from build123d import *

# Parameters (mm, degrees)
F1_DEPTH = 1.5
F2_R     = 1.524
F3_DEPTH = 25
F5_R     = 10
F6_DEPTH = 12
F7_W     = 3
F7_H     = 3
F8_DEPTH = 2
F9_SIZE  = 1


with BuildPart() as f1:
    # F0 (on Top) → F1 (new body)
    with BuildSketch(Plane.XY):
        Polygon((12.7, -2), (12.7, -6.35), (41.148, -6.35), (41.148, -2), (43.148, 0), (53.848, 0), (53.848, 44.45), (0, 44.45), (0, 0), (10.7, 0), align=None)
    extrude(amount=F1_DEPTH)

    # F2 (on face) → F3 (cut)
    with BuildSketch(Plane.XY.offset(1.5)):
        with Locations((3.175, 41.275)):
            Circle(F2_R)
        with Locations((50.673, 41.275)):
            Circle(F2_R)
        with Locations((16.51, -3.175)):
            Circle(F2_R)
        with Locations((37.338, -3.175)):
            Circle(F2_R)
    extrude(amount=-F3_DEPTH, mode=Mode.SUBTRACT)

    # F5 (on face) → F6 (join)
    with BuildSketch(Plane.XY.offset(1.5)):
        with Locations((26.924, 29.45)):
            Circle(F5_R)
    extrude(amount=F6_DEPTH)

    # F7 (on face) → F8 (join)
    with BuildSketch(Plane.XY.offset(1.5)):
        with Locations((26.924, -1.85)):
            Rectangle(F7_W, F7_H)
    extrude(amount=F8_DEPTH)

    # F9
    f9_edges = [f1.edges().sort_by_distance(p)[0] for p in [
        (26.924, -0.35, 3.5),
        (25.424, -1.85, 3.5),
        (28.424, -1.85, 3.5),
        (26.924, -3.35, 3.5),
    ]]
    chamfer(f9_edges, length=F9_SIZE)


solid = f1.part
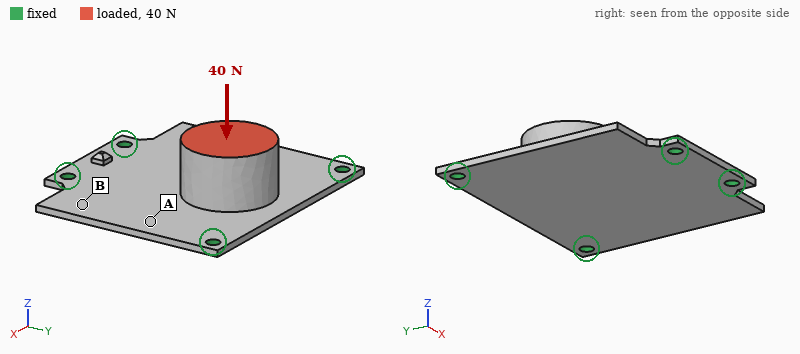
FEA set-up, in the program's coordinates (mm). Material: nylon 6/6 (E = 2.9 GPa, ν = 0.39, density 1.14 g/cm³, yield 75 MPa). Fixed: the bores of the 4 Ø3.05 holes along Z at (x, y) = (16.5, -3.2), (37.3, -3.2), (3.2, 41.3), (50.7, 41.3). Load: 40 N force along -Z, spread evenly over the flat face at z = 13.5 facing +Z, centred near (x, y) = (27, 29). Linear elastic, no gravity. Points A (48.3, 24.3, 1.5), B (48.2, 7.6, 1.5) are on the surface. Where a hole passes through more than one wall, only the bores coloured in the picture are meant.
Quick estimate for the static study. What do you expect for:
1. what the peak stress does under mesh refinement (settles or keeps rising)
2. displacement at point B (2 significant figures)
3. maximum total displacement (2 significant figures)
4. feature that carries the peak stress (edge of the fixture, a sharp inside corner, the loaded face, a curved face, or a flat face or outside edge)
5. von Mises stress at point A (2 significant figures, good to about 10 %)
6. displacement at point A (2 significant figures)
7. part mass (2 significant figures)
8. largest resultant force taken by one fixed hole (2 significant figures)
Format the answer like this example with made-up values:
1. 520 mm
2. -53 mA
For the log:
1. keeps rising
2. 0.098 mm
3. 0.43 mm
4. edge of the fixture
5. 4.3 MPa
6. 0.23 mm
7. 8.7 g
8. 16 N
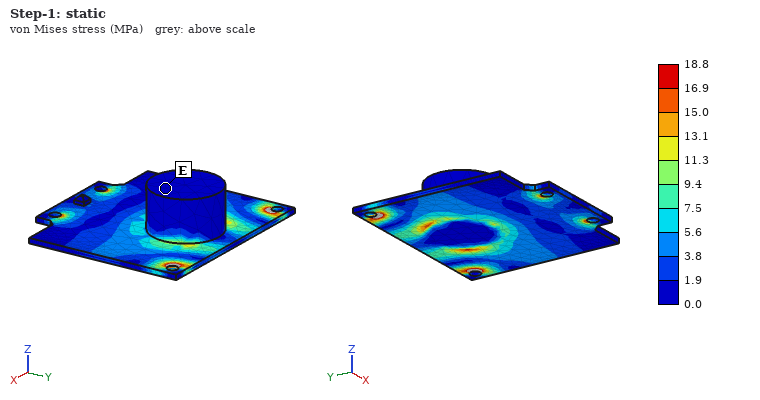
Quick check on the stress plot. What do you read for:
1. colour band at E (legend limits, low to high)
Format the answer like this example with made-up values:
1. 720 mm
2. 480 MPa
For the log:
1. 0.0 to 1.9 MPa
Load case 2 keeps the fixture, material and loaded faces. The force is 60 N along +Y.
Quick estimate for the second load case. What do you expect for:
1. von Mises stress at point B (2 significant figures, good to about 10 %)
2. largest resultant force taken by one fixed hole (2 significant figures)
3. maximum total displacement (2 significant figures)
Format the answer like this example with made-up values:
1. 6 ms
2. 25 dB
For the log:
1. 2.5 MPa
2. 21 N
3. 0.71 mm
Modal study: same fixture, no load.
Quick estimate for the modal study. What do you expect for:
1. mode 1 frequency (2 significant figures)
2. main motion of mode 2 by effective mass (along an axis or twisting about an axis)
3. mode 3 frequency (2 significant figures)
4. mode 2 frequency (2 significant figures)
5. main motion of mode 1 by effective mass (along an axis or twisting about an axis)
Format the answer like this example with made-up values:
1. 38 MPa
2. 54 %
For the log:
1. 630 Hz
2. along Y
3. 1000 Hz
4. 940 Hz
5. along Z
